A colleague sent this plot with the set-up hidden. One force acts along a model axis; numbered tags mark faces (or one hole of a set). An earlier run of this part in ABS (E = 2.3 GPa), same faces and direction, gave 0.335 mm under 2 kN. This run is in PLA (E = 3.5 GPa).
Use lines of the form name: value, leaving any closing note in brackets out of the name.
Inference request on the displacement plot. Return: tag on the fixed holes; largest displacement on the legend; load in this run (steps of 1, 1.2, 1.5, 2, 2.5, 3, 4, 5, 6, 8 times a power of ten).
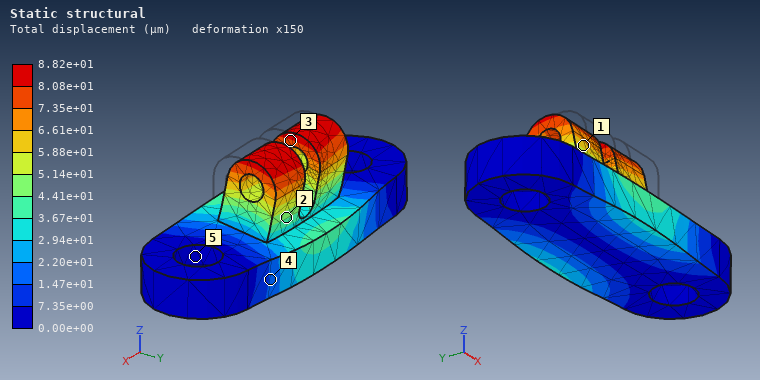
tag on the fixed holes: 5
largest displacement on the legend: 8.82e+01 µm
load in this run: 800 N
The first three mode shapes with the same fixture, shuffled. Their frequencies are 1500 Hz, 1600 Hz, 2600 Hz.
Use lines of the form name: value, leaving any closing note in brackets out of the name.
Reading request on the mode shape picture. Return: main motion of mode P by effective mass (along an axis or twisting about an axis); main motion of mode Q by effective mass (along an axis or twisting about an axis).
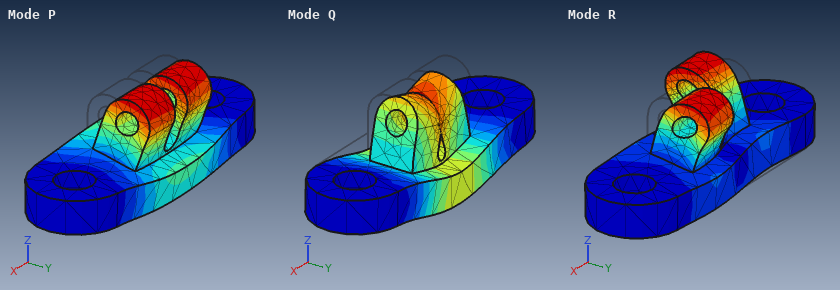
main motion of mode P by effective mass: along Y
main motion of mode Q by effective mass: along Z
